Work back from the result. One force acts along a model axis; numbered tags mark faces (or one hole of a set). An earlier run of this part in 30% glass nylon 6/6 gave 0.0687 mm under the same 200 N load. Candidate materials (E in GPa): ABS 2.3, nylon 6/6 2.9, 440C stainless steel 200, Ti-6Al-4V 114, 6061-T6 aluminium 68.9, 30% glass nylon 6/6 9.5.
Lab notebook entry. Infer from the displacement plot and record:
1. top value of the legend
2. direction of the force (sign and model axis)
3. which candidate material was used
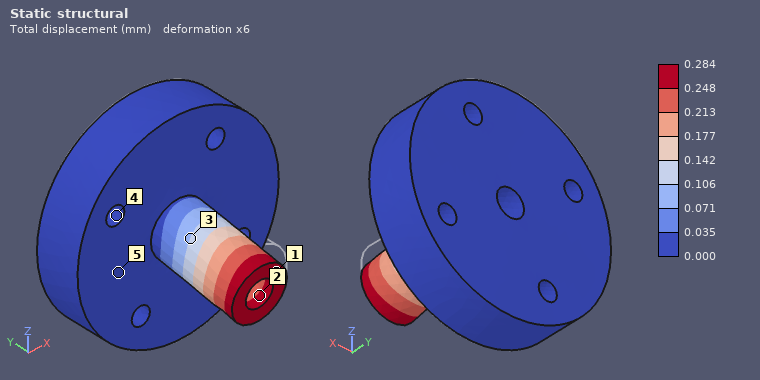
0.284 mm
-Z
ABS
